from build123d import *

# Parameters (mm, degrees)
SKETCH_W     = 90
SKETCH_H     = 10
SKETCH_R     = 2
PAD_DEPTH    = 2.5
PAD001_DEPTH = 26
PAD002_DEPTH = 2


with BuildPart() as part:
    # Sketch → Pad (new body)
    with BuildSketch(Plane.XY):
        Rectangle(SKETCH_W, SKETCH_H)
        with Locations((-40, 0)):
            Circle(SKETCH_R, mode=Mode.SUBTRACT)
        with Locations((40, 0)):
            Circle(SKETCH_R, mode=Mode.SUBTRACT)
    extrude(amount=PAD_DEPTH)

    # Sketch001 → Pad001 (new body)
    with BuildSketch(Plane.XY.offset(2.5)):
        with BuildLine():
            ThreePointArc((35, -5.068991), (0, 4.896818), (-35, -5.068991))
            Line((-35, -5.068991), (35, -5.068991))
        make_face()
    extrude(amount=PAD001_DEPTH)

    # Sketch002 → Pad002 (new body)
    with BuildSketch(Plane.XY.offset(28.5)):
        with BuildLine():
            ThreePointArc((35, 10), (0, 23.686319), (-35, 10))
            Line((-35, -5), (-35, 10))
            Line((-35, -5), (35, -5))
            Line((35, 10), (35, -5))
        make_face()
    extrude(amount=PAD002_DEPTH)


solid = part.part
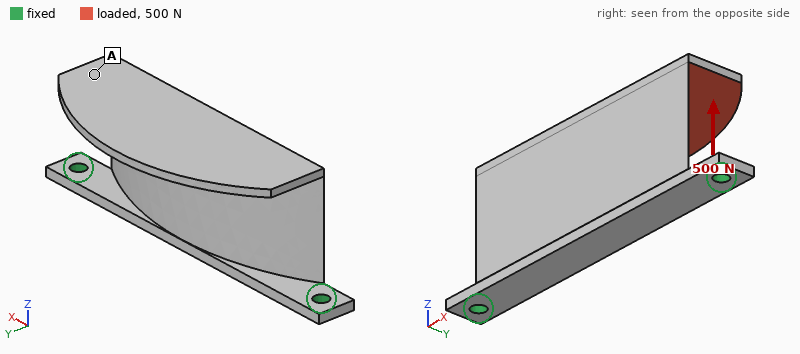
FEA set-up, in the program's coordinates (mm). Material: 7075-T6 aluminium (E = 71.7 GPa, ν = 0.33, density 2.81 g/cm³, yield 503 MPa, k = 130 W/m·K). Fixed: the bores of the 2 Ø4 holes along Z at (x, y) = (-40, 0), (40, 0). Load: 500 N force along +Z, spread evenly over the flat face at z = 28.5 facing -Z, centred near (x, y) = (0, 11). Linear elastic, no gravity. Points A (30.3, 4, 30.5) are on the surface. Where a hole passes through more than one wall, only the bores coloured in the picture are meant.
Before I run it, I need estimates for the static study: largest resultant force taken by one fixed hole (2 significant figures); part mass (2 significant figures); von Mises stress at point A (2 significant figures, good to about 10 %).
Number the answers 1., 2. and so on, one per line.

1. 290 N
2. 50 g
3. 26 MPa
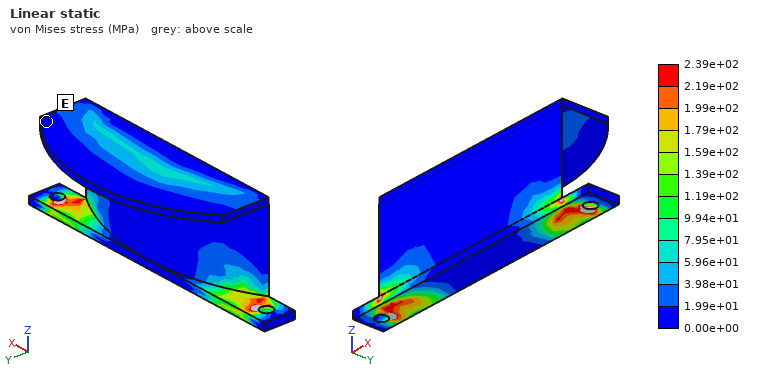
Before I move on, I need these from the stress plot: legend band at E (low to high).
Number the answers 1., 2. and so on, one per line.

1. 0.00e+00 to 1.99e+01 MPa
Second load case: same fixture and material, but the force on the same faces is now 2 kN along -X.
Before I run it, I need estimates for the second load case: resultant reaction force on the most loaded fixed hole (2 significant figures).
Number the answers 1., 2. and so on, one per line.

1. 1.3 kN
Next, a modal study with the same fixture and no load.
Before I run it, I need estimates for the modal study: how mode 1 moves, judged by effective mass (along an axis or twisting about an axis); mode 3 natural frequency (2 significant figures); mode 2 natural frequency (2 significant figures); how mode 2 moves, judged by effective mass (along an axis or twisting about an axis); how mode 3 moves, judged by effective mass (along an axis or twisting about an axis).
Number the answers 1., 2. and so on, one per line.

1. along Y
2. 4000 Hz
3. 3000 Hz
4. along Z
5. along X
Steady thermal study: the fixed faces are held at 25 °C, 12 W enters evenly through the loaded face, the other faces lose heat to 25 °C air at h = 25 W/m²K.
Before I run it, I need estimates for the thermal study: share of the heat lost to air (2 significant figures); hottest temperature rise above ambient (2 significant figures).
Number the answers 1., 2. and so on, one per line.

1. 30 %
2. 29 K
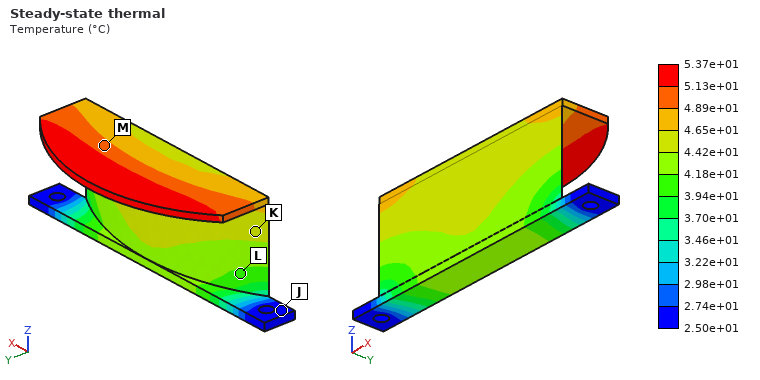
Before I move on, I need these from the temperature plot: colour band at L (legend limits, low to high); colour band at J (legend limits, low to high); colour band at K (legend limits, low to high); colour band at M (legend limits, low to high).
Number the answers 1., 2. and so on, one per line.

1. 3.94e+01 to 4.18e+01 °C
2. 2.50e+01 to 2.74e+01 °C
3. 4.42e+01 to 4.65e+01 °C
4. 4.89e+01 to 5.13e+01 °C
